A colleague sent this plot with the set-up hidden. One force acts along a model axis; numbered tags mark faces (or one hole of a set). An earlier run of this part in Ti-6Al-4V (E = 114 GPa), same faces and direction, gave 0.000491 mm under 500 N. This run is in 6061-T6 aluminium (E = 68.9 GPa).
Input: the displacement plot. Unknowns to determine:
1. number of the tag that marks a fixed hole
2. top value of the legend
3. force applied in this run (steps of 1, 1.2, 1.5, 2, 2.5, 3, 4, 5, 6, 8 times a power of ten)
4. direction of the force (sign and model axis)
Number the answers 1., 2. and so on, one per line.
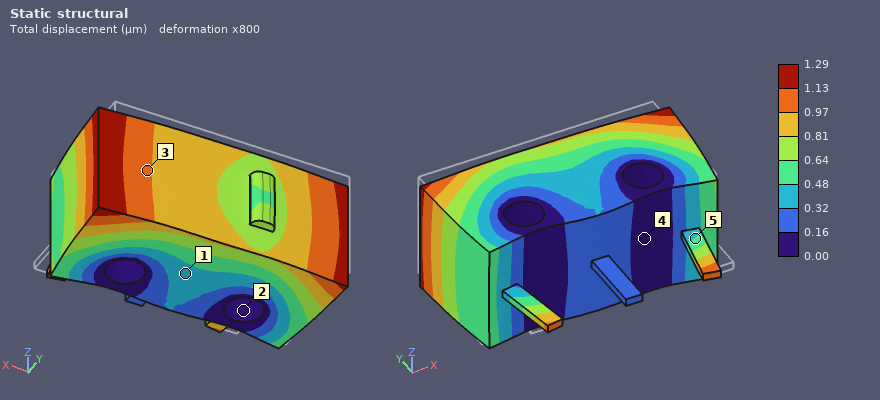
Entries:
1. 2
2. 1.29 µm
3. 800 N
4. -Y
